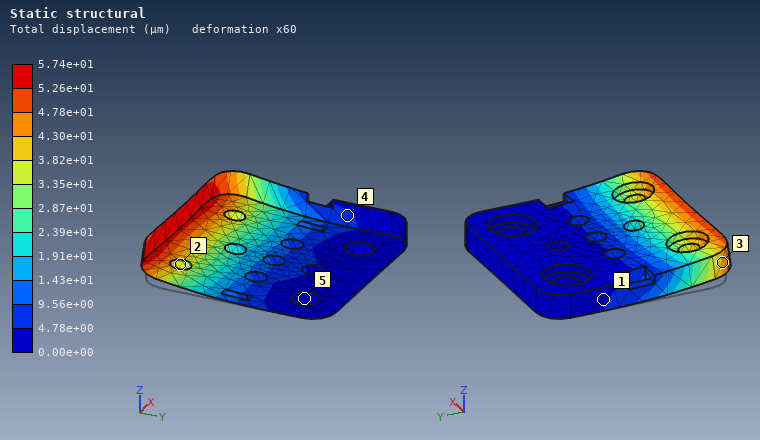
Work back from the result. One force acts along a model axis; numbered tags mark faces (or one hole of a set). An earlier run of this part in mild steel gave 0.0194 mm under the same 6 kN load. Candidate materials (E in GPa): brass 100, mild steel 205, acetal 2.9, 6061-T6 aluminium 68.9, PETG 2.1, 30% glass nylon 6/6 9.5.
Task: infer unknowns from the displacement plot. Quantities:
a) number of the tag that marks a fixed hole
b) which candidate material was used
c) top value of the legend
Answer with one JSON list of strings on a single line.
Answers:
["5", "6061-T6 aluminium", "5.74e+01 µm"]
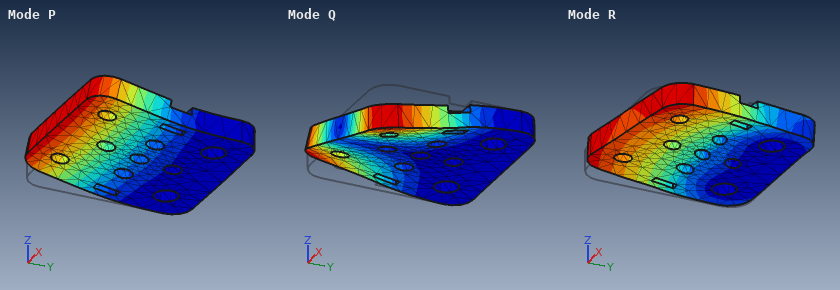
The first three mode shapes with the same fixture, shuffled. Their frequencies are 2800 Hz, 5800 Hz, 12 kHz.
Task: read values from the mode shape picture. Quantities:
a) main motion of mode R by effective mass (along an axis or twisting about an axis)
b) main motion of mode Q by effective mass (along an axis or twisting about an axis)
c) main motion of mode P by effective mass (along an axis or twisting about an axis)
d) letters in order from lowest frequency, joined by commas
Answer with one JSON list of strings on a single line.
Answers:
["along X", "twisting about Y", "along Z", "P, Q, R"]
